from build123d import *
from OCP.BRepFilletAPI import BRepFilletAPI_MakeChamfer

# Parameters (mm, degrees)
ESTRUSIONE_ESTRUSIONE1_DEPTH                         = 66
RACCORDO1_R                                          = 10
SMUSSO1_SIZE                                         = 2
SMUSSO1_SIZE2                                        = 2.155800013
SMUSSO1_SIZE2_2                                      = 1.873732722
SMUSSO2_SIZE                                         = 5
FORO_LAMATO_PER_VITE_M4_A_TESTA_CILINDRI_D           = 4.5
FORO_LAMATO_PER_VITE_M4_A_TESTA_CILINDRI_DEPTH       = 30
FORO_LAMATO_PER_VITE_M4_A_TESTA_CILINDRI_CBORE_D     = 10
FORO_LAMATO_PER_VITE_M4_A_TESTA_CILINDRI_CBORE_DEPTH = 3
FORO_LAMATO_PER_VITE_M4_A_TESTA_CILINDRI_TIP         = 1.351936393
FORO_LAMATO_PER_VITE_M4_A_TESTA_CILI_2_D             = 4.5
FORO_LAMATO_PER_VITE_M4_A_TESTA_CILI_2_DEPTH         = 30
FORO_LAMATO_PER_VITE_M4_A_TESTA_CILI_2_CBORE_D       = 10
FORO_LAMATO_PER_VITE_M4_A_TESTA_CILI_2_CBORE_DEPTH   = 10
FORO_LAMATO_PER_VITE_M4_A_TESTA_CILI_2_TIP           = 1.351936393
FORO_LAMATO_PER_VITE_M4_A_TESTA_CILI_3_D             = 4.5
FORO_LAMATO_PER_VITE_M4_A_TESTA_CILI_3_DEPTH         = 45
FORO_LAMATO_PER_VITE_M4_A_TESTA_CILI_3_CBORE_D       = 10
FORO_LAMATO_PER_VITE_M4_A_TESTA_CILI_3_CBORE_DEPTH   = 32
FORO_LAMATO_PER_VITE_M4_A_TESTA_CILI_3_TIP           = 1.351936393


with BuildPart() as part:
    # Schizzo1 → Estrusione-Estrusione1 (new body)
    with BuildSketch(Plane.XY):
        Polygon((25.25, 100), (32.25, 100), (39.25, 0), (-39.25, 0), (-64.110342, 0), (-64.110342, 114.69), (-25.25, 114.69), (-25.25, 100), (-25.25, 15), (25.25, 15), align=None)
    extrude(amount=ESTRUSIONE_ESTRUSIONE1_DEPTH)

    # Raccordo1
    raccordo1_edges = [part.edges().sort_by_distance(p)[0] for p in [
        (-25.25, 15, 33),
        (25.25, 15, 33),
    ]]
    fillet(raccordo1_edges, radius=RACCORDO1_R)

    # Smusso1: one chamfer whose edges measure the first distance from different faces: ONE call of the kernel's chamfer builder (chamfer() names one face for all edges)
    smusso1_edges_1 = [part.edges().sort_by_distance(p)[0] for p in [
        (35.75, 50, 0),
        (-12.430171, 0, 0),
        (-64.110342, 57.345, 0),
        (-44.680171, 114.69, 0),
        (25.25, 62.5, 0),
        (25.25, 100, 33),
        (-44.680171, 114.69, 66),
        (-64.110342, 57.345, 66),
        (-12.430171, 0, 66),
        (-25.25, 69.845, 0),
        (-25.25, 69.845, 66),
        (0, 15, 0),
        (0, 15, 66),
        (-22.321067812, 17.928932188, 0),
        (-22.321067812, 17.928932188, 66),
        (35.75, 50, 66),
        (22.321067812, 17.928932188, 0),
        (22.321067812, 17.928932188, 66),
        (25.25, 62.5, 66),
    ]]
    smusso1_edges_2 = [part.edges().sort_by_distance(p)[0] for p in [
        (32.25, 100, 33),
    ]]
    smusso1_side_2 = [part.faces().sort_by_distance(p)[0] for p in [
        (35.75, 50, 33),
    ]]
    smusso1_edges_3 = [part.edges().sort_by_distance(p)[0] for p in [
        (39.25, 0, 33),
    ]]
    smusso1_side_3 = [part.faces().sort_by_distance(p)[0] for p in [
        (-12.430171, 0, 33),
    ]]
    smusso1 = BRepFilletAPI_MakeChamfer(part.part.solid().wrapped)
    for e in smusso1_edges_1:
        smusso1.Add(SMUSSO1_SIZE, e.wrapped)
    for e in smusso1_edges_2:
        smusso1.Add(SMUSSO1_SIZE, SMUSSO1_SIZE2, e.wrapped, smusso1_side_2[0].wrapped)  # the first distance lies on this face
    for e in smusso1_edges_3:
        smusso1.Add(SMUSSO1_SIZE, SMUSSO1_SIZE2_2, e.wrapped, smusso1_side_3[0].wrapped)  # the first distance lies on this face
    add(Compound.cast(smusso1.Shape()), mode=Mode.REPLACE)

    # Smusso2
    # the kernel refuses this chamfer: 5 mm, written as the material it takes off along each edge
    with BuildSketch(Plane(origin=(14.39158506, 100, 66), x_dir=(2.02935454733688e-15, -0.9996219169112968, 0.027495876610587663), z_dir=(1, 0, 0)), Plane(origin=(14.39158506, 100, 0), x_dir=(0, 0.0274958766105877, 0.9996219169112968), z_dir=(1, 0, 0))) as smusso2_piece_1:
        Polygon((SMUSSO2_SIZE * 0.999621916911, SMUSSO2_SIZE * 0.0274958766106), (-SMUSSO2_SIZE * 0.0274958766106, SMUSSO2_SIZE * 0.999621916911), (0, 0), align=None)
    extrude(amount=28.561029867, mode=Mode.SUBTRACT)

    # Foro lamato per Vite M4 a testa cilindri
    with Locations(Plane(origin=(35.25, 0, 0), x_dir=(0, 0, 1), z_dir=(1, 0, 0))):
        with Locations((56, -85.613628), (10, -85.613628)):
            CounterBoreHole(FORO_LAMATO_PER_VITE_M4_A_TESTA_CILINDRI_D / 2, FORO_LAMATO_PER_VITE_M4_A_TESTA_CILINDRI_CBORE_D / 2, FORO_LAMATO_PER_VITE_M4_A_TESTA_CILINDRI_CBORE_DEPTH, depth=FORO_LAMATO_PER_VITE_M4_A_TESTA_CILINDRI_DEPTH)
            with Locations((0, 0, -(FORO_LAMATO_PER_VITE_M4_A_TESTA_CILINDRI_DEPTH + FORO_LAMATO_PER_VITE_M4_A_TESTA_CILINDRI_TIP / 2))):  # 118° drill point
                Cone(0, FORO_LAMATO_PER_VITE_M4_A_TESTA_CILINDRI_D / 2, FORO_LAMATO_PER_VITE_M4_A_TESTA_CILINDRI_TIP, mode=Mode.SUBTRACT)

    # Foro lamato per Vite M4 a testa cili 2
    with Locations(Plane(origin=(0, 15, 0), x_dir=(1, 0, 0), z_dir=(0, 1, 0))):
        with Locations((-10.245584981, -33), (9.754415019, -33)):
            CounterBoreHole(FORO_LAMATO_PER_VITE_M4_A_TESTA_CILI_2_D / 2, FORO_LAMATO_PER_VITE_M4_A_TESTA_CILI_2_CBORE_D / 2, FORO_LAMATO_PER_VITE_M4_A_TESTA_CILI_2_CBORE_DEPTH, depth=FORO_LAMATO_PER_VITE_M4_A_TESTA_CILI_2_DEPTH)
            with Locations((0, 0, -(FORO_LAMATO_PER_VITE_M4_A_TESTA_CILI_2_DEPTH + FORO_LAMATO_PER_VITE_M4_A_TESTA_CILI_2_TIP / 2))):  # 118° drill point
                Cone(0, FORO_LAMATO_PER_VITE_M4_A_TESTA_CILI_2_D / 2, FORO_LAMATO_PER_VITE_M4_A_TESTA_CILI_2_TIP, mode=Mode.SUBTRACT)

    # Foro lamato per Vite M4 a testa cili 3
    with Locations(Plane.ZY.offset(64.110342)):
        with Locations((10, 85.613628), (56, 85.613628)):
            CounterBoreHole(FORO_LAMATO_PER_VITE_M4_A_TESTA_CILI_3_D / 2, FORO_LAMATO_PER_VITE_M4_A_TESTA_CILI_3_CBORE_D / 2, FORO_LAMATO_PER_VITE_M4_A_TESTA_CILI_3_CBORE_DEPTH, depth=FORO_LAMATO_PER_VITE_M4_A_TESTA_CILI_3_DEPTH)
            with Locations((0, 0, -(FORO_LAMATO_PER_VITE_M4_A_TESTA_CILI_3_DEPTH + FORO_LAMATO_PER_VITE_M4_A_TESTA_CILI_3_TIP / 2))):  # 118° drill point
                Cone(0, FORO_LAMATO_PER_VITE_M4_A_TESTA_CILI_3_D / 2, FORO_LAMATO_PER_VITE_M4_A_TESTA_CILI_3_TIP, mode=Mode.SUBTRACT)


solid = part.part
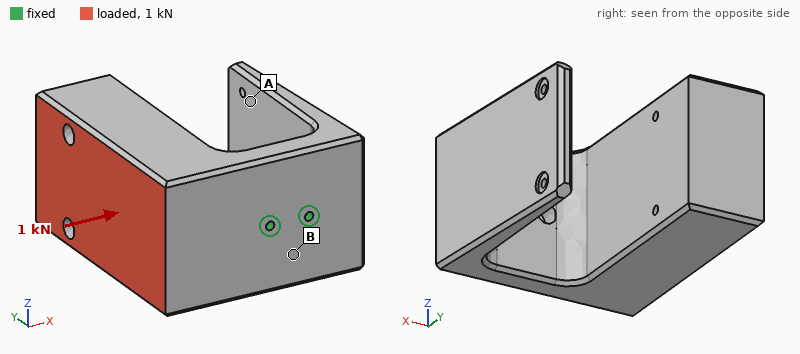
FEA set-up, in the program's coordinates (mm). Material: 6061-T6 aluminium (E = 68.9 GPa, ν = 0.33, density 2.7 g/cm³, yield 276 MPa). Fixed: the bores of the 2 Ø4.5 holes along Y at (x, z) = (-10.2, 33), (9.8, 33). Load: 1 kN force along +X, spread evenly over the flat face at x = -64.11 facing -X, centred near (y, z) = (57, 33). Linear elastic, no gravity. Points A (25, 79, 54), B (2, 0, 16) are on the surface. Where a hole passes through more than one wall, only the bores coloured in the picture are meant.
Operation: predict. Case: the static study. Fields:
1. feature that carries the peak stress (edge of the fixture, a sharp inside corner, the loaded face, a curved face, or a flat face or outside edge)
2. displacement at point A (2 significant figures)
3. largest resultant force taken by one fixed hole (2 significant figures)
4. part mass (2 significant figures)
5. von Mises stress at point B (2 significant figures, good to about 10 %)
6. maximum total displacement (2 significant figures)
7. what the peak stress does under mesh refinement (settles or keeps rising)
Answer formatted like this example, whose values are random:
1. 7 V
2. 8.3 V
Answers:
1. edge of the fixture
2. 0.042 mm
3. 2.5 kN
4. 1.1 kg
5. 6.6 MPa
6. 0.19 mm
7. keeps rising
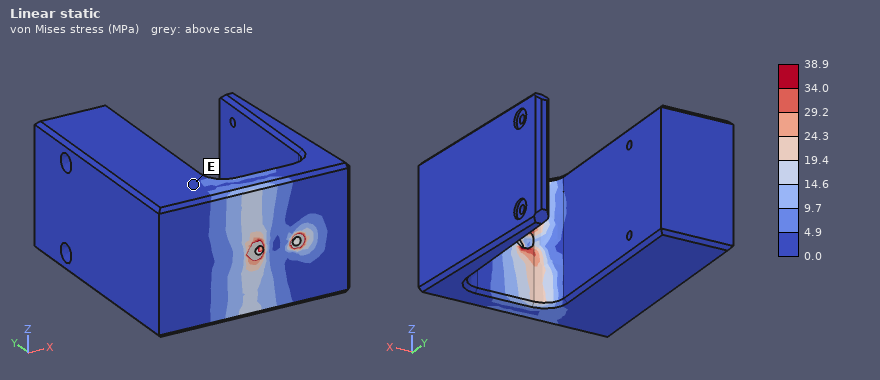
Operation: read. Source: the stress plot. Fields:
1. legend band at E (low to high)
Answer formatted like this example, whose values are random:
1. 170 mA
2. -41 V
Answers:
1. 0.0 to 4.9 MPa
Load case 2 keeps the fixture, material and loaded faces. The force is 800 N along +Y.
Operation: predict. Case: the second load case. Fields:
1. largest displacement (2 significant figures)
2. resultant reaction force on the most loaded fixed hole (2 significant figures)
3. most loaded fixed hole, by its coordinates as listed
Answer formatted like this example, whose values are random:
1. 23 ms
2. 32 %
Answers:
1. 0.15 mm
2. 2.6 kN
3. (-10.2, 33)
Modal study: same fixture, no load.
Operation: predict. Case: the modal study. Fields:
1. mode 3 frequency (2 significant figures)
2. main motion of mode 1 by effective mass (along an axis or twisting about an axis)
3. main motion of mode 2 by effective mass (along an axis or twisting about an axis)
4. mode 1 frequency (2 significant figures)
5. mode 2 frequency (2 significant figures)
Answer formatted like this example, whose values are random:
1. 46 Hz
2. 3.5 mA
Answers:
1. 1100 Hz
2. along Z
3. along X
4. 280 Hz
5. 460 Hz
